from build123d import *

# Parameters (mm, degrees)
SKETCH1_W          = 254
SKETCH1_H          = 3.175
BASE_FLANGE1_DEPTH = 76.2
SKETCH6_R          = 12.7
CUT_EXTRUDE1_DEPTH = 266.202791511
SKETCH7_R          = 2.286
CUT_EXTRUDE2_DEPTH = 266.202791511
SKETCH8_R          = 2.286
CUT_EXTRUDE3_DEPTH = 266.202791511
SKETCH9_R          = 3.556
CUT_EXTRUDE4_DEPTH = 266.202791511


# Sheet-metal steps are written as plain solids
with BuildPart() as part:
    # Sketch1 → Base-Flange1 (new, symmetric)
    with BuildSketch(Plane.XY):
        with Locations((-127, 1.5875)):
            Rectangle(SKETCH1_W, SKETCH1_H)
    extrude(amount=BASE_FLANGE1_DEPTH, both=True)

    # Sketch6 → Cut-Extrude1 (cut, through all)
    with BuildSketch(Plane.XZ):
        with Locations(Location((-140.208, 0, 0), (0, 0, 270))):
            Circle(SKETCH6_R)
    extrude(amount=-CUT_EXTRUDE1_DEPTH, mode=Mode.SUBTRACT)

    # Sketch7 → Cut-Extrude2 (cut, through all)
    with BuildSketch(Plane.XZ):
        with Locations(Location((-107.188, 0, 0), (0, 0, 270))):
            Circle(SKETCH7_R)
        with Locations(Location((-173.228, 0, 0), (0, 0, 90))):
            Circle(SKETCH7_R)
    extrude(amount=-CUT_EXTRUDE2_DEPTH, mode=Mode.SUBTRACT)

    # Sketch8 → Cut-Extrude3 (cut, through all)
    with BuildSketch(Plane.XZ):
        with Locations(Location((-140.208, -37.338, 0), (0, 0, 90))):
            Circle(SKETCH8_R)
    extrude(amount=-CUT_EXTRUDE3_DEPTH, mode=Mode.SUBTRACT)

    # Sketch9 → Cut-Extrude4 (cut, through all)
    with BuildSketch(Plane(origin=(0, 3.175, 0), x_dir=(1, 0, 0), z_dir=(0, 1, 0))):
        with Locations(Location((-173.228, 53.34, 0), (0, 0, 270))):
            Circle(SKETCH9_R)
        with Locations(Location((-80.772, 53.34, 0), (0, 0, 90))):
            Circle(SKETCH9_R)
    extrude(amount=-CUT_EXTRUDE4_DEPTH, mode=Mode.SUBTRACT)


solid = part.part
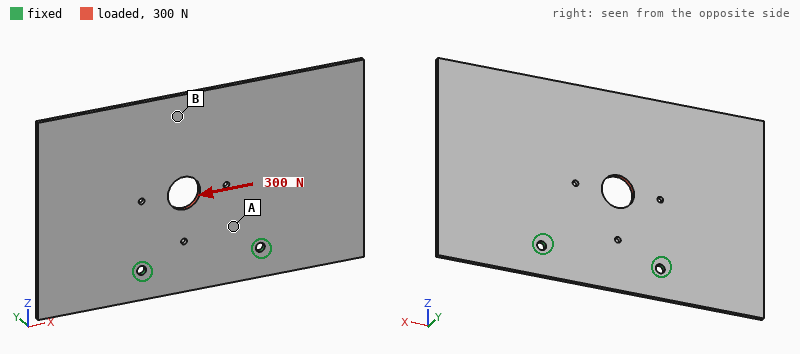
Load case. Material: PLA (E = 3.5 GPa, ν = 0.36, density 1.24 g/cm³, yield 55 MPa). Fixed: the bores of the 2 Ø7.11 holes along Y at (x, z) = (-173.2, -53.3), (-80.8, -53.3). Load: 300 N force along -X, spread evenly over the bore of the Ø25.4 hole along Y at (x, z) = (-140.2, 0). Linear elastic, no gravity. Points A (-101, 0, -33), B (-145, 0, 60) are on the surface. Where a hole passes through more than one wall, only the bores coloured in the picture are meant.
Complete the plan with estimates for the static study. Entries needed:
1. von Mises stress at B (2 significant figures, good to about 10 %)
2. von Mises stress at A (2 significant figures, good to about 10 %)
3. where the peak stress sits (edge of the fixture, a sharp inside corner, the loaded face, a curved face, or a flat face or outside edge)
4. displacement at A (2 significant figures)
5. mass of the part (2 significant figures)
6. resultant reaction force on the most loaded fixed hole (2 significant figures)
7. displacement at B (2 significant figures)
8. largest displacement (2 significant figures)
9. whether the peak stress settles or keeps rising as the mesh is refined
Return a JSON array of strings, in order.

["0.33 MPa", "1.5 MPa", "edge of the fixture", "0.019 mm", "150 g", "230 N", "0.076 mm", "0.11 mm", "keeps rising"]
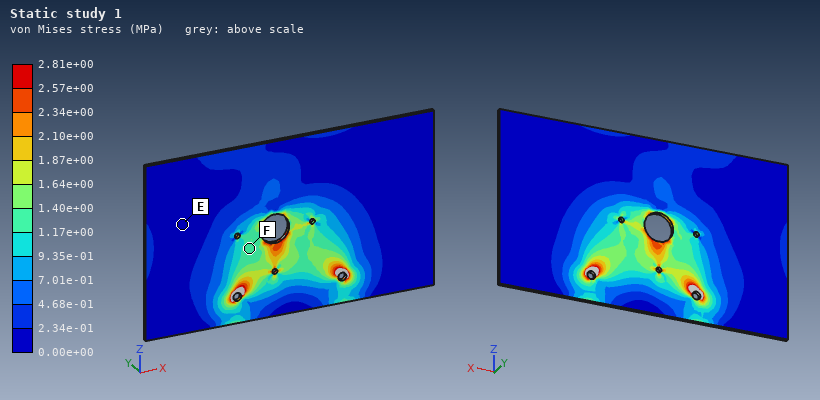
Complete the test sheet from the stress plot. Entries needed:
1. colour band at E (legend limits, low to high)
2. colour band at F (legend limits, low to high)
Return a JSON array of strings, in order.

["0.00e+00 to 2.34e-01 MPa", "1.17e+00 to 1.40e+00 MPa"]
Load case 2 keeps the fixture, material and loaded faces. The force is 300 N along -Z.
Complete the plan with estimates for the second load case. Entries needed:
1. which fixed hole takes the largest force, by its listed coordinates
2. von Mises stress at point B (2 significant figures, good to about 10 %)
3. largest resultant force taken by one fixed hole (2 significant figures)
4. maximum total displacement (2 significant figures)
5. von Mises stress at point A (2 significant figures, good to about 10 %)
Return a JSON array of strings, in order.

["(-173.2, -53.3)", "0.33 MPa", "190 N", "30 µm", "0.76 MPa"]
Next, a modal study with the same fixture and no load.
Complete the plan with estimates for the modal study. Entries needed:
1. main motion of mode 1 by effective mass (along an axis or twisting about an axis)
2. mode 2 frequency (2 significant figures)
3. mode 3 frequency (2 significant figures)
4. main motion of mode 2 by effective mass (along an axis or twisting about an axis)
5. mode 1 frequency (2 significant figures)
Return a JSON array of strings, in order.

["along Y", "58 Hz", "100 Hz", "twisting about Z", "43 Hz"]
